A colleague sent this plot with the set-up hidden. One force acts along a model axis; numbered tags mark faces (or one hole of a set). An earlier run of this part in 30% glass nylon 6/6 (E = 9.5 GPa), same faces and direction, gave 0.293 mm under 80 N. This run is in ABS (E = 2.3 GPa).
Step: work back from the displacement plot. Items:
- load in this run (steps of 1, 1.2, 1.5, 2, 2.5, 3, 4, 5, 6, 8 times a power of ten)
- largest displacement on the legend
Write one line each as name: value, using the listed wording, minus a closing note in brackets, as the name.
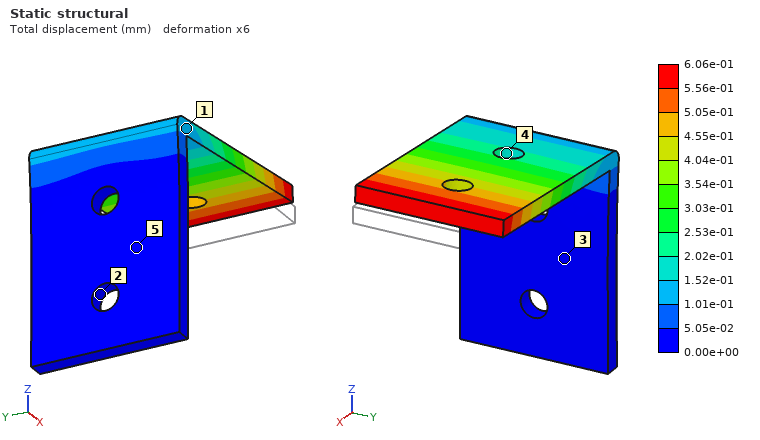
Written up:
load in this run: 40 N
largest displacement on the legend: 6.06e-01 mm
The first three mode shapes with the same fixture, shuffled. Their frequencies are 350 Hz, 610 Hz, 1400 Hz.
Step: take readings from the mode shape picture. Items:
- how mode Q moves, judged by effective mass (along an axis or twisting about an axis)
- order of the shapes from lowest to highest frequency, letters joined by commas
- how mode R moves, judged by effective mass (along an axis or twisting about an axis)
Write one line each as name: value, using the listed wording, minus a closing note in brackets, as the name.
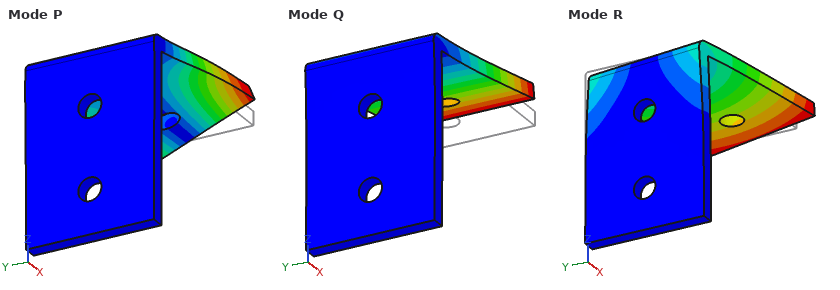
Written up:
how mode Q moves, judged by effective mass: along Z
order of the shapes from lowest to highest frequency, letters joined by commas: Q, R, P
how mode R moves, judged by effective mass: along Y
